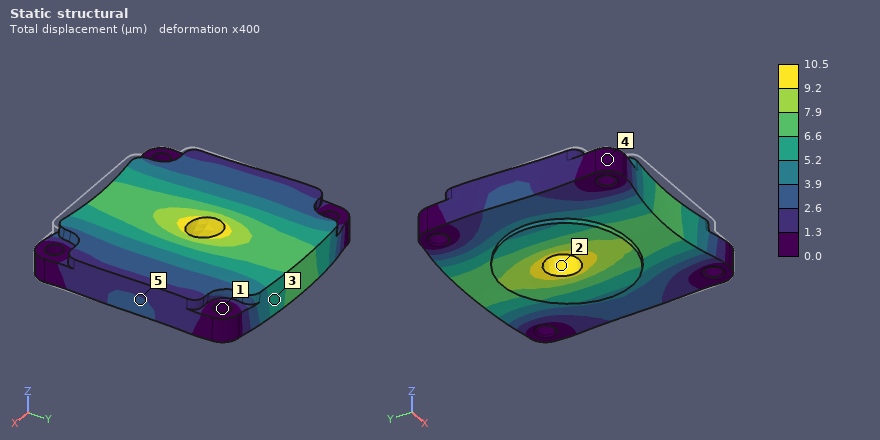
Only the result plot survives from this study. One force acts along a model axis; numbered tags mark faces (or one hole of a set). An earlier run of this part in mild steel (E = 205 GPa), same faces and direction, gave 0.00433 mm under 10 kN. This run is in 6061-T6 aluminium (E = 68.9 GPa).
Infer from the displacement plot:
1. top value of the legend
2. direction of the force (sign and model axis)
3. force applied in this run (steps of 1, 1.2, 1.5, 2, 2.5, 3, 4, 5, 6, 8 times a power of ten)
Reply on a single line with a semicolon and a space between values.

10.5 µm; +Y; 8 kN
